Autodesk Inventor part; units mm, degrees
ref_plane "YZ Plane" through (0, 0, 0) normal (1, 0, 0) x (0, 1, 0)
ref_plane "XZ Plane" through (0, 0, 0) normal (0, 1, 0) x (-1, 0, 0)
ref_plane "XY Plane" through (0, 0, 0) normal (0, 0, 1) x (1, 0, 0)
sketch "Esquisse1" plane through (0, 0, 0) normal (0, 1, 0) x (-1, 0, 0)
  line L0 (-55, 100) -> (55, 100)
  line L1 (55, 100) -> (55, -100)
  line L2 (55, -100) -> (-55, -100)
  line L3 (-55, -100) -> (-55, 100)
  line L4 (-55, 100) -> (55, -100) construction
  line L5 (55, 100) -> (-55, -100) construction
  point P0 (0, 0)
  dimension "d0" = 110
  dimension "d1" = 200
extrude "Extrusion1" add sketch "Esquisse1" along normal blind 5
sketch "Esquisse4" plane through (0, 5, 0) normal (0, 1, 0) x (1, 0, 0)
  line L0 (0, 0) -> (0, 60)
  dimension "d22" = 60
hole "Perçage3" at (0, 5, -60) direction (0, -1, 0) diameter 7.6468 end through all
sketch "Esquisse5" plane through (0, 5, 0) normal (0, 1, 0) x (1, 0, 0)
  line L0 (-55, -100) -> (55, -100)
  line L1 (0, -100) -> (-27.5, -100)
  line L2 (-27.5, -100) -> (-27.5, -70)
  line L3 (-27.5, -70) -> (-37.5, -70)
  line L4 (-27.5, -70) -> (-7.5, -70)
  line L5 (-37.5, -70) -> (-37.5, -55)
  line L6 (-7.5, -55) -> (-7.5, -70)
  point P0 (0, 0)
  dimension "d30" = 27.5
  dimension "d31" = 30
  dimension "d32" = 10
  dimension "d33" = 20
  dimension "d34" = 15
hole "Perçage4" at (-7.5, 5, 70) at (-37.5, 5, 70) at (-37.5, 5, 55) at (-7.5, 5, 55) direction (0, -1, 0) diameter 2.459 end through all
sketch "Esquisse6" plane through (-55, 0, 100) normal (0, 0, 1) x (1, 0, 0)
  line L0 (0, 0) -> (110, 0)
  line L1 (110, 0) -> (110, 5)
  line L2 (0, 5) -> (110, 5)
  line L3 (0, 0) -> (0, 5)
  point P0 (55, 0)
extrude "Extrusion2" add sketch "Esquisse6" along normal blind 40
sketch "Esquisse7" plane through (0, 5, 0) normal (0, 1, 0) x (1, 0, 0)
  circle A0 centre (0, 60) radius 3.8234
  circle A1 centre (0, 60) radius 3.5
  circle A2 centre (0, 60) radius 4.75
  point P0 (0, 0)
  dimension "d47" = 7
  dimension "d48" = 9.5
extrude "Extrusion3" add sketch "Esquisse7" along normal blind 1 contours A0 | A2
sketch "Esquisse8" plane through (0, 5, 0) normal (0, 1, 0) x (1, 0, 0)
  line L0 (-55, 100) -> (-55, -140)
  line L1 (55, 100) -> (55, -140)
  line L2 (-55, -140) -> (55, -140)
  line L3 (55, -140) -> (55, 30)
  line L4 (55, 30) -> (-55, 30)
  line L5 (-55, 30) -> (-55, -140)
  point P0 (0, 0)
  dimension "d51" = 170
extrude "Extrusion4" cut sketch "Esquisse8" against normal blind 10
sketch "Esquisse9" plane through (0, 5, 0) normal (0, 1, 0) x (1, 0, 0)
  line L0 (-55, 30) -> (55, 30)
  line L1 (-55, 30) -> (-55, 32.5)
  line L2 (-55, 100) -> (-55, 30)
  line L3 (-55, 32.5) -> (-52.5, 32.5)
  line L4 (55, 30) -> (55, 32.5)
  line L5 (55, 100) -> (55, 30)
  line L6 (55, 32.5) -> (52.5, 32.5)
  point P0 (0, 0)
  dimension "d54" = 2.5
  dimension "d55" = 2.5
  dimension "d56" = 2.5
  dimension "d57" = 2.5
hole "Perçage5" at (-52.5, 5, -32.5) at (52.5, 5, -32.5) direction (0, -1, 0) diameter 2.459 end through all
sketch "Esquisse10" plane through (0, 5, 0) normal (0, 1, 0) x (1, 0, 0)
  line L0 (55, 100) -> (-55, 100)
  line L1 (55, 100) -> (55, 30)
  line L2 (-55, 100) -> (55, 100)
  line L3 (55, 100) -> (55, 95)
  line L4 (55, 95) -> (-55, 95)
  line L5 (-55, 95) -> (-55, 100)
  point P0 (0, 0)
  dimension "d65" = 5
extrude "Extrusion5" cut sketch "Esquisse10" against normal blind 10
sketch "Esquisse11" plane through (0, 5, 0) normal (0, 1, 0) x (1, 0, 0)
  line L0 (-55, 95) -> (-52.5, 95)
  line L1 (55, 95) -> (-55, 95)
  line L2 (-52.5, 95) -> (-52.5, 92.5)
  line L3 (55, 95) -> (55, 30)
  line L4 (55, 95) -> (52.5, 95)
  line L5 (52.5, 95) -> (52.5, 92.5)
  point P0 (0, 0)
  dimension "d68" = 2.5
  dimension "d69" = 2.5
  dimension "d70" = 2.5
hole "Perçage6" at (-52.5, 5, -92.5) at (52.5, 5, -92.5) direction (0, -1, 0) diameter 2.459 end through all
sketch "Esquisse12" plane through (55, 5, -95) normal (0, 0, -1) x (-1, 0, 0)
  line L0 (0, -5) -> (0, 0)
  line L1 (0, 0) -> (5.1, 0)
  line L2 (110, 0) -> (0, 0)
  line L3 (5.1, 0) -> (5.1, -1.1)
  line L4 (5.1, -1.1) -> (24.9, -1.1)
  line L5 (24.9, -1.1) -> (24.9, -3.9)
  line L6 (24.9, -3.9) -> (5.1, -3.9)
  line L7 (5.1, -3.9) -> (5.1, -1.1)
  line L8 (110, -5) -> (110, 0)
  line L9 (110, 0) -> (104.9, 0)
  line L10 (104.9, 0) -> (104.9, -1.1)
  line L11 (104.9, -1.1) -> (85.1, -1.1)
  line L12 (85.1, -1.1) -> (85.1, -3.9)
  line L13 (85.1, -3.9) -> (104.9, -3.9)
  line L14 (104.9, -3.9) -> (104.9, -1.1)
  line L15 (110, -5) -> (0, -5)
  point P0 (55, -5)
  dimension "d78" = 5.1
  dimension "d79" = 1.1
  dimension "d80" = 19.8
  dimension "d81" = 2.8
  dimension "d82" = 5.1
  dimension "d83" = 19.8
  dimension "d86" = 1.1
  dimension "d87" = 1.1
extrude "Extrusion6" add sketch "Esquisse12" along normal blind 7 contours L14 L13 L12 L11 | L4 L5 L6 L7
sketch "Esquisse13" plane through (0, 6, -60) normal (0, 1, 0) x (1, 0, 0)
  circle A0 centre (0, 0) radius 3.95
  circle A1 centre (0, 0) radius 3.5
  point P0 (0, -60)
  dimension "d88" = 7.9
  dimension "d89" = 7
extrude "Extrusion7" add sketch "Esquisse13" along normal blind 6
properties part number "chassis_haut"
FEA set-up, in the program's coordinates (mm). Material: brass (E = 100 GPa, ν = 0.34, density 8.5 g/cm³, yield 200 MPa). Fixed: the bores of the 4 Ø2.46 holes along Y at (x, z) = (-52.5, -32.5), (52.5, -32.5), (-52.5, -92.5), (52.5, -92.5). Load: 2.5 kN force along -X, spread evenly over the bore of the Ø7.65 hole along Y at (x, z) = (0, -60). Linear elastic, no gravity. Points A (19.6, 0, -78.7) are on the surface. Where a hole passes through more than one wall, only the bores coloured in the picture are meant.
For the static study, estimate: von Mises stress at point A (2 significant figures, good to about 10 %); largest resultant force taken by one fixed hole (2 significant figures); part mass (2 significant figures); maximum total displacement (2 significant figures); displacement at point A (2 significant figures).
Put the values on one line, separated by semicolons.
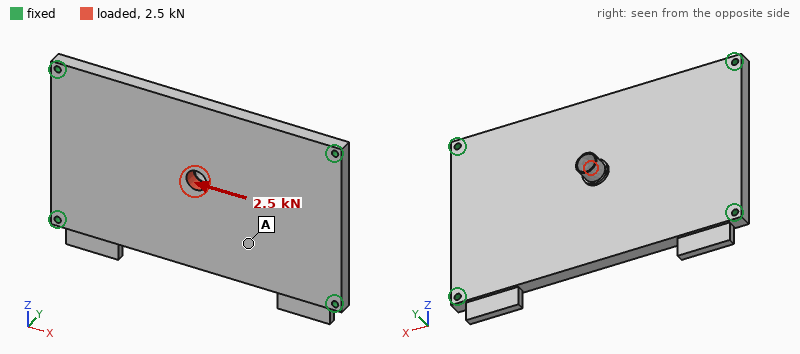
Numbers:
5.1 MPa; 680 N; 310 g; 5.9 µm; 3.0 µm
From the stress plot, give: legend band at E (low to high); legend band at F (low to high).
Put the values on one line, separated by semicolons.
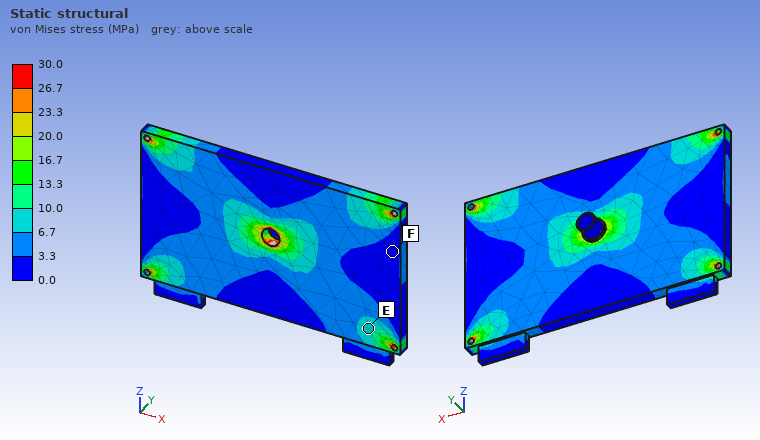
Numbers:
6.7 to 10.0 MPa; 0.0 to 3.3 MPa
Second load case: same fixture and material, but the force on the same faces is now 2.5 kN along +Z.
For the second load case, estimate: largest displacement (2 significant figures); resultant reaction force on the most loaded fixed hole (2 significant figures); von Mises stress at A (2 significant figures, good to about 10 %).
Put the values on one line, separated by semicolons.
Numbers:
9.9 µm; 840 N; 7.9 MPa
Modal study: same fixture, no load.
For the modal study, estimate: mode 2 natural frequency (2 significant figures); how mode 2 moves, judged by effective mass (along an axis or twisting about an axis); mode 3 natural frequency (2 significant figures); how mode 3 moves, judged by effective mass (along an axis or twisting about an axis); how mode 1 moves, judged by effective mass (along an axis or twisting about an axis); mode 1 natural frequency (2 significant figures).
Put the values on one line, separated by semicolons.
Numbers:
2100 Hz; twisting about X; 3100 Hz; twisting about Z; along Y; 1100 Hz
